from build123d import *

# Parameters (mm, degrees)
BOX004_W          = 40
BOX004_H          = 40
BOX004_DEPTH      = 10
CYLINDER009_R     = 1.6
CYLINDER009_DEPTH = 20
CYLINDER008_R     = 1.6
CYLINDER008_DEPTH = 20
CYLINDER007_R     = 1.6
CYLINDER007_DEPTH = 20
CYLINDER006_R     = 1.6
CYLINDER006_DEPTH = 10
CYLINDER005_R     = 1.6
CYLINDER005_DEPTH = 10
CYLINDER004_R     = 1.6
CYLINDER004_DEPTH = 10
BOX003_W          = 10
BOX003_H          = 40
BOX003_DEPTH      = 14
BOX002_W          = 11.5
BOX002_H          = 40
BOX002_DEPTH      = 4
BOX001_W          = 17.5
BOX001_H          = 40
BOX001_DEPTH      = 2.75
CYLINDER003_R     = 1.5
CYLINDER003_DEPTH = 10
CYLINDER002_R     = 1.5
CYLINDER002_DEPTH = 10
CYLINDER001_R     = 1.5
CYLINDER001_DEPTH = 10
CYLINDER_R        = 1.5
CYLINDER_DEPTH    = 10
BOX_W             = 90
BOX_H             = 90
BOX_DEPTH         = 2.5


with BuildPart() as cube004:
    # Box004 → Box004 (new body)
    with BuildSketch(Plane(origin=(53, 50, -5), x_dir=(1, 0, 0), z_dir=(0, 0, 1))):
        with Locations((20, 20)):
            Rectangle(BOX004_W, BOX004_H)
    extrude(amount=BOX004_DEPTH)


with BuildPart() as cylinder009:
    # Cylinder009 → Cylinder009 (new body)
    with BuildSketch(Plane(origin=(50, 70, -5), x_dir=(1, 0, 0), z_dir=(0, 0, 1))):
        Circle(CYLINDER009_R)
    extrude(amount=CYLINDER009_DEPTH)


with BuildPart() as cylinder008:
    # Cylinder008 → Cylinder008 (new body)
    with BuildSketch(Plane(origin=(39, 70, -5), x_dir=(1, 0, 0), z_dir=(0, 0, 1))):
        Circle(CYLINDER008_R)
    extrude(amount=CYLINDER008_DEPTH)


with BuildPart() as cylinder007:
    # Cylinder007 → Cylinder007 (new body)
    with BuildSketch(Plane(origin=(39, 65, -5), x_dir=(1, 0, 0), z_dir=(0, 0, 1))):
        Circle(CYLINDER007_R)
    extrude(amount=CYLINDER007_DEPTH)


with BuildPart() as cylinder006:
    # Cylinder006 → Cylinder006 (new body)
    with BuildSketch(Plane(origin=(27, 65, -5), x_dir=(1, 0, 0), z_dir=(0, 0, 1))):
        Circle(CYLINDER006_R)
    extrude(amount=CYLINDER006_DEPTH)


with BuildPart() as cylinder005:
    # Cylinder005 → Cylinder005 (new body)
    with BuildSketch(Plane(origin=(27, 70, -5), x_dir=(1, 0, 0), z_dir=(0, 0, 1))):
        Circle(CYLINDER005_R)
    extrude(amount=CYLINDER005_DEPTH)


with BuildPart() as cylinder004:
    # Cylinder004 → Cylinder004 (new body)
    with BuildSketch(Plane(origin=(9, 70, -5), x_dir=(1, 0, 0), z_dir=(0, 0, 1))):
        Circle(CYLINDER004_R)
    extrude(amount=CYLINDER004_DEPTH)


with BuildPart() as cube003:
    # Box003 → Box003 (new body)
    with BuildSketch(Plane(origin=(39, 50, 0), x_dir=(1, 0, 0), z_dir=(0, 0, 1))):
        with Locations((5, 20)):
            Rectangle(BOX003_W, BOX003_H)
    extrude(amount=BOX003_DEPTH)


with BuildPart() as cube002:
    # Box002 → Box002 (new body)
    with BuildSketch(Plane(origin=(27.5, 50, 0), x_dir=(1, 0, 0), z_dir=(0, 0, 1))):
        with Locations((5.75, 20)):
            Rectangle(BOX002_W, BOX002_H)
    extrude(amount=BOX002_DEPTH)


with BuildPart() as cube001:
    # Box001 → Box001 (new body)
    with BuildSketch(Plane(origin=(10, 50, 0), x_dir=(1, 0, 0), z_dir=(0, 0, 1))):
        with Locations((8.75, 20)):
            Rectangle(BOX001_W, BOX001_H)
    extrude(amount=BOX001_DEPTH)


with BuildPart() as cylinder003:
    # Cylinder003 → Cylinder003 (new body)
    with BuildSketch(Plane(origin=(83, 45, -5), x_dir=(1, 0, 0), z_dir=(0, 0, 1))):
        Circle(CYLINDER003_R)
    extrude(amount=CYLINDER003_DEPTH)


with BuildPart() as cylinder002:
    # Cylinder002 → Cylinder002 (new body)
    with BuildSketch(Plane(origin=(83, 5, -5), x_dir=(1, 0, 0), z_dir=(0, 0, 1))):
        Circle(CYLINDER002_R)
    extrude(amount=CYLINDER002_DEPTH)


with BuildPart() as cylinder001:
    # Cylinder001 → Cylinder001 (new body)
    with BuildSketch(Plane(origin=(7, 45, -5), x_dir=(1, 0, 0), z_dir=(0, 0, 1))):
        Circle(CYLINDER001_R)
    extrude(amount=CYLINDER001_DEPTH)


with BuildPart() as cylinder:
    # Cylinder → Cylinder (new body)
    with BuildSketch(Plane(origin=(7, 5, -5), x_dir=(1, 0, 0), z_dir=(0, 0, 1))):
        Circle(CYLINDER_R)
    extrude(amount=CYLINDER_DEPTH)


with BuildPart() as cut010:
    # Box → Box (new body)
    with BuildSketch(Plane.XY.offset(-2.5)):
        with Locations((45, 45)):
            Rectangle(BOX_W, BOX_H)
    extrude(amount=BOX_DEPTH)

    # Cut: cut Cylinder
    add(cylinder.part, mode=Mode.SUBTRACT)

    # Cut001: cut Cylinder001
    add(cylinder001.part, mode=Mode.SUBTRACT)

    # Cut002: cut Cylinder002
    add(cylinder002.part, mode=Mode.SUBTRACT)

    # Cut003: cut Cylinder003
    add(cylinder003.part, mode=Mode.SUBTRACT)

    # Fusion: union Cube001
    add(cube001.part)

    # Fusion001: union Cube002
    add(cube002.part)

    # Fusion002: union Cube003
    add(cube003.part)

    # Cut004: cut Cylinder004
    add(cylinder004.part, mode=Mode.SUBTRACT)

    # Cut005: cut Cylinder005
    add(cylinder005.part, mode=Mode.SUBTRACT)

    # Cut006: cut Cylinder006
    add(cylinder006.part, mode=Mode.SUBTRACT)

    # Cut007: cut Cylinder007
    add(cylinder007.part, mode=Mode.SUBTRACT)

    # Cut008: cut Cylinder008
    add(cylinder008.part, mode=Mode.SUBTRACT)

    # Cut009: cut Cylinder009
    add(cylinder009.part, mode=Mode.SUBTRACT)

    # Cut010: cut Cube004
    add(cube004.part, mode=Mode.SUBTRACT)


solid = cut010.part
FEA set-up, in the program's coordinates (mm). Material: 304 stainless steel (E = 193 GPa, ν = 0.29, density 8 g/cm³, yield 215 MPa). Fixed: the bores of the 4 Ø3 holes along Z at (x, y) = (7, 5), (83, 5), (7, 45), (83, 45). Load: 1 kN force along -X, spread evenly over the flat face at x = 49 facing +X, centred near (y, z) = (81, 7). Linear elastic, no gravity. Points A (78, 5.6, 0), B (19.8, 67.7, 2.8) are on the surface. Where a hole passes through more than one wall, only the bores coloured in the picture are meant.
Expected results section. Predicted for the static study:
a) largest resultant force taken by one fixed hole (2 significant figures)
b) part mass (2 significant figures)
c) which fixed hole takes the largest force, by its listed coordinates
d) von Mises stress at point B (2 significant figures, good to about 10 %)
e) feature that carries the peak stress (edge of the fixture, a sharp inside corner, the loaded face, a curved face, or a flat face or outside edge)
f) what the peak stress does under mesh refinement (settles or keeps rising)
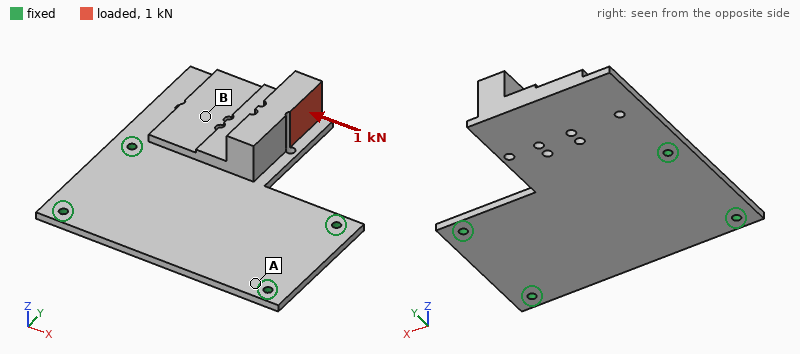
1.1 kN
200 g
(7, 45)
22 MPa
edge of the fixture
keeps rising
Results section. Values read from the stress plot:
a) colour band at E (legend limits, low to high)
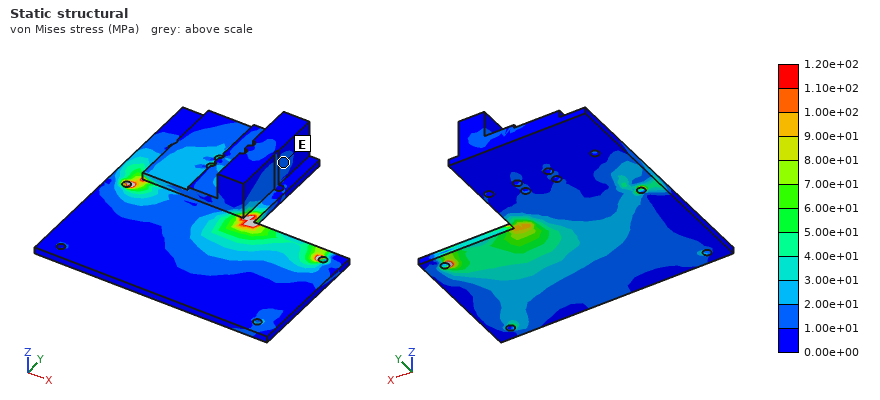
1.00e+01 to 2.00e+01 MPa
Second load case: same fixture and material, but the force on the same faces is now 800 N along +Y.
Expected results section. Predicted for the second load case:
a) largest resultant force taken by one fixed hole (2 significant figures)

330 N
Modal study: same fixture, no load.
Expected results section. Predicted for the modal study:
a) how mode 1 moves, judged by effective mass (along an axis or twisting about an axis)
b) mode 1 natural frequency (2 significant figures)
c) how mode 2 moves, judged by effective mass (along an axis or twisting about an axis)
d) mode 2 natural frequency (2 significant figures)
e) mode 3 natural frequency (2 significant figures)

along Z
520 Hz
along Z
1600 Hz
2600 Hz
